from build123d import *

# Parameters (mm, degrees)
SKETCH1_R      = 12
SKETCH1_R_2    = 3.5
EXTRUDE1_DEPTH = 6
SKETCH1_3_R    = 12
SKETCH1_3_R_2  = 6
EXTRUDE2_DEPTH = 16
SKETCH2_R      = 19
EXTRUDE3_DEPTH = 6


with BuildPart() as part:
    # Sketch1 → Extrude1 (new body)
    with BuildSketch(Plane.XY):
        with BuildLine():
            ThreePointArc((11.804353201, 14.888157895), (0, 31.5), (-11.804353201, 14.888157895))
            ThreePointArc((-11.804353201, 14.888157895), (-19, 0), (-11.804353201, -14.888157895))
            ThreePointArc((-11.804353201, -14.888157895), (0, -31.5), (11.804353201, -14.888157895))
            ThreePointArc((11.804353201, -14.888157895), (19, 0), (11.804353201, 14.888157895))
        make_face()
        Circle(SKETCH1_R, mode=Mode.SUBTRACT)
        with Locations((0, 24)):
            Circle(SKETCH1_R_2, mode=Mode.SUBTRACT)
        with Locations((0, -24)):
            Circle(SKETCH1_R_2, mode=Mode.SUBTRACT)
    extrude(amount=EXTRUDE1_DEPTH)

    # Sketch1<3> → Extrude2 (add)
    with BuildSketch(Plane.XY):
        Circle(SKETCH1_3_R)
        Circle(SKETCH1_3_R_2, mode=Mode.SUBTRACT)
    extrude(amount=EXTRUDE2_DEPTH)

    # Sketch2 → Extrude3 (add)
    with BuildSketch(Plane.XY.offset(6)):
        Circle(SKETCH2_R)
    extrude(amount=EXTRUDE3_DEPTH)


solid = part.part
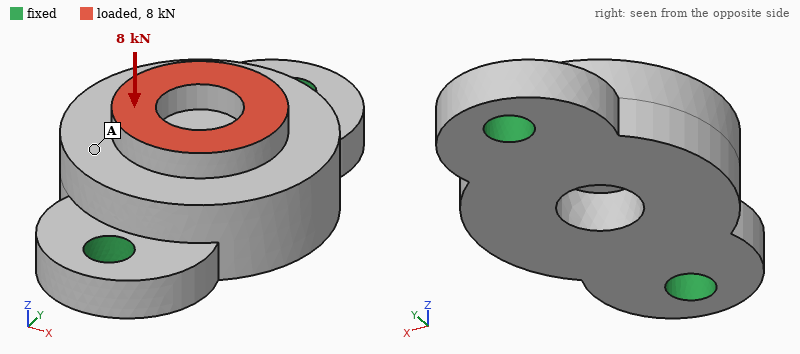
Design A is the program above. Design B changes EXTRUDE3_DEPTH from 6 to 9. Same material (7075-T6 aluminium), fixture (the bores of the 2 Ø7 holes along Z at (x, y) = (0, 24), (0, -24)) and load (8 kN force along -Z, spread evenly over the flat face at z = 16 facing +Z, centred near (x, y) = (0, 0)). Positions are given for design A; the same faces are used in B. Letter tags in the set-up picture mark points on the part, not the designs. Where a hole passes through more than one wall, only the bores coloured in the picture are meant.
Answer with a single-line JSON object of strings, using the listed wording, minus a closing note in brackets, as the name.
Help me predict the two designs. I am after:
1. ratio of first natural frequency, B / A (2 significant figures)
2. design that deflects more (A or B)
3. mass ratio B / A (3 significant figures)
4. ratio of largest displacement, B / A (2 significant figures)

{"ratio of first natural frequency, B / A": "0.90", "design that deflects more": "A", "mass ratio B / A": "1.14", "ratio of largest displacement, B / A": "0.79"}
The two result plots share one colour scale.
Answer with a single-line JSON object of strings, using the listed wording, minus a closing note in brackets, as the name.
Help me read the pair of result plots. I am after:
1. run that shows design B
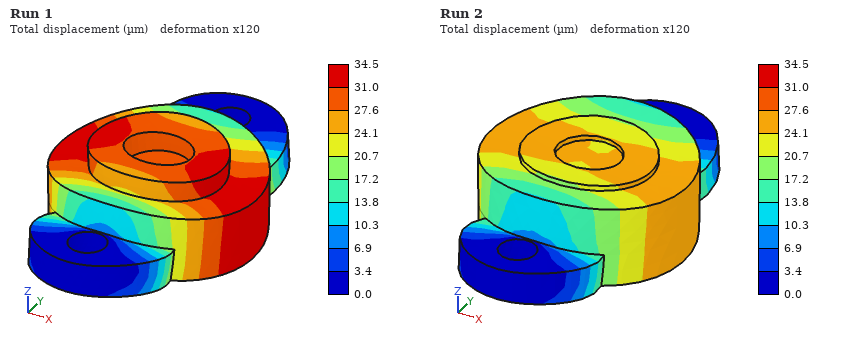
{"run that shows design B": "Run 2"}
